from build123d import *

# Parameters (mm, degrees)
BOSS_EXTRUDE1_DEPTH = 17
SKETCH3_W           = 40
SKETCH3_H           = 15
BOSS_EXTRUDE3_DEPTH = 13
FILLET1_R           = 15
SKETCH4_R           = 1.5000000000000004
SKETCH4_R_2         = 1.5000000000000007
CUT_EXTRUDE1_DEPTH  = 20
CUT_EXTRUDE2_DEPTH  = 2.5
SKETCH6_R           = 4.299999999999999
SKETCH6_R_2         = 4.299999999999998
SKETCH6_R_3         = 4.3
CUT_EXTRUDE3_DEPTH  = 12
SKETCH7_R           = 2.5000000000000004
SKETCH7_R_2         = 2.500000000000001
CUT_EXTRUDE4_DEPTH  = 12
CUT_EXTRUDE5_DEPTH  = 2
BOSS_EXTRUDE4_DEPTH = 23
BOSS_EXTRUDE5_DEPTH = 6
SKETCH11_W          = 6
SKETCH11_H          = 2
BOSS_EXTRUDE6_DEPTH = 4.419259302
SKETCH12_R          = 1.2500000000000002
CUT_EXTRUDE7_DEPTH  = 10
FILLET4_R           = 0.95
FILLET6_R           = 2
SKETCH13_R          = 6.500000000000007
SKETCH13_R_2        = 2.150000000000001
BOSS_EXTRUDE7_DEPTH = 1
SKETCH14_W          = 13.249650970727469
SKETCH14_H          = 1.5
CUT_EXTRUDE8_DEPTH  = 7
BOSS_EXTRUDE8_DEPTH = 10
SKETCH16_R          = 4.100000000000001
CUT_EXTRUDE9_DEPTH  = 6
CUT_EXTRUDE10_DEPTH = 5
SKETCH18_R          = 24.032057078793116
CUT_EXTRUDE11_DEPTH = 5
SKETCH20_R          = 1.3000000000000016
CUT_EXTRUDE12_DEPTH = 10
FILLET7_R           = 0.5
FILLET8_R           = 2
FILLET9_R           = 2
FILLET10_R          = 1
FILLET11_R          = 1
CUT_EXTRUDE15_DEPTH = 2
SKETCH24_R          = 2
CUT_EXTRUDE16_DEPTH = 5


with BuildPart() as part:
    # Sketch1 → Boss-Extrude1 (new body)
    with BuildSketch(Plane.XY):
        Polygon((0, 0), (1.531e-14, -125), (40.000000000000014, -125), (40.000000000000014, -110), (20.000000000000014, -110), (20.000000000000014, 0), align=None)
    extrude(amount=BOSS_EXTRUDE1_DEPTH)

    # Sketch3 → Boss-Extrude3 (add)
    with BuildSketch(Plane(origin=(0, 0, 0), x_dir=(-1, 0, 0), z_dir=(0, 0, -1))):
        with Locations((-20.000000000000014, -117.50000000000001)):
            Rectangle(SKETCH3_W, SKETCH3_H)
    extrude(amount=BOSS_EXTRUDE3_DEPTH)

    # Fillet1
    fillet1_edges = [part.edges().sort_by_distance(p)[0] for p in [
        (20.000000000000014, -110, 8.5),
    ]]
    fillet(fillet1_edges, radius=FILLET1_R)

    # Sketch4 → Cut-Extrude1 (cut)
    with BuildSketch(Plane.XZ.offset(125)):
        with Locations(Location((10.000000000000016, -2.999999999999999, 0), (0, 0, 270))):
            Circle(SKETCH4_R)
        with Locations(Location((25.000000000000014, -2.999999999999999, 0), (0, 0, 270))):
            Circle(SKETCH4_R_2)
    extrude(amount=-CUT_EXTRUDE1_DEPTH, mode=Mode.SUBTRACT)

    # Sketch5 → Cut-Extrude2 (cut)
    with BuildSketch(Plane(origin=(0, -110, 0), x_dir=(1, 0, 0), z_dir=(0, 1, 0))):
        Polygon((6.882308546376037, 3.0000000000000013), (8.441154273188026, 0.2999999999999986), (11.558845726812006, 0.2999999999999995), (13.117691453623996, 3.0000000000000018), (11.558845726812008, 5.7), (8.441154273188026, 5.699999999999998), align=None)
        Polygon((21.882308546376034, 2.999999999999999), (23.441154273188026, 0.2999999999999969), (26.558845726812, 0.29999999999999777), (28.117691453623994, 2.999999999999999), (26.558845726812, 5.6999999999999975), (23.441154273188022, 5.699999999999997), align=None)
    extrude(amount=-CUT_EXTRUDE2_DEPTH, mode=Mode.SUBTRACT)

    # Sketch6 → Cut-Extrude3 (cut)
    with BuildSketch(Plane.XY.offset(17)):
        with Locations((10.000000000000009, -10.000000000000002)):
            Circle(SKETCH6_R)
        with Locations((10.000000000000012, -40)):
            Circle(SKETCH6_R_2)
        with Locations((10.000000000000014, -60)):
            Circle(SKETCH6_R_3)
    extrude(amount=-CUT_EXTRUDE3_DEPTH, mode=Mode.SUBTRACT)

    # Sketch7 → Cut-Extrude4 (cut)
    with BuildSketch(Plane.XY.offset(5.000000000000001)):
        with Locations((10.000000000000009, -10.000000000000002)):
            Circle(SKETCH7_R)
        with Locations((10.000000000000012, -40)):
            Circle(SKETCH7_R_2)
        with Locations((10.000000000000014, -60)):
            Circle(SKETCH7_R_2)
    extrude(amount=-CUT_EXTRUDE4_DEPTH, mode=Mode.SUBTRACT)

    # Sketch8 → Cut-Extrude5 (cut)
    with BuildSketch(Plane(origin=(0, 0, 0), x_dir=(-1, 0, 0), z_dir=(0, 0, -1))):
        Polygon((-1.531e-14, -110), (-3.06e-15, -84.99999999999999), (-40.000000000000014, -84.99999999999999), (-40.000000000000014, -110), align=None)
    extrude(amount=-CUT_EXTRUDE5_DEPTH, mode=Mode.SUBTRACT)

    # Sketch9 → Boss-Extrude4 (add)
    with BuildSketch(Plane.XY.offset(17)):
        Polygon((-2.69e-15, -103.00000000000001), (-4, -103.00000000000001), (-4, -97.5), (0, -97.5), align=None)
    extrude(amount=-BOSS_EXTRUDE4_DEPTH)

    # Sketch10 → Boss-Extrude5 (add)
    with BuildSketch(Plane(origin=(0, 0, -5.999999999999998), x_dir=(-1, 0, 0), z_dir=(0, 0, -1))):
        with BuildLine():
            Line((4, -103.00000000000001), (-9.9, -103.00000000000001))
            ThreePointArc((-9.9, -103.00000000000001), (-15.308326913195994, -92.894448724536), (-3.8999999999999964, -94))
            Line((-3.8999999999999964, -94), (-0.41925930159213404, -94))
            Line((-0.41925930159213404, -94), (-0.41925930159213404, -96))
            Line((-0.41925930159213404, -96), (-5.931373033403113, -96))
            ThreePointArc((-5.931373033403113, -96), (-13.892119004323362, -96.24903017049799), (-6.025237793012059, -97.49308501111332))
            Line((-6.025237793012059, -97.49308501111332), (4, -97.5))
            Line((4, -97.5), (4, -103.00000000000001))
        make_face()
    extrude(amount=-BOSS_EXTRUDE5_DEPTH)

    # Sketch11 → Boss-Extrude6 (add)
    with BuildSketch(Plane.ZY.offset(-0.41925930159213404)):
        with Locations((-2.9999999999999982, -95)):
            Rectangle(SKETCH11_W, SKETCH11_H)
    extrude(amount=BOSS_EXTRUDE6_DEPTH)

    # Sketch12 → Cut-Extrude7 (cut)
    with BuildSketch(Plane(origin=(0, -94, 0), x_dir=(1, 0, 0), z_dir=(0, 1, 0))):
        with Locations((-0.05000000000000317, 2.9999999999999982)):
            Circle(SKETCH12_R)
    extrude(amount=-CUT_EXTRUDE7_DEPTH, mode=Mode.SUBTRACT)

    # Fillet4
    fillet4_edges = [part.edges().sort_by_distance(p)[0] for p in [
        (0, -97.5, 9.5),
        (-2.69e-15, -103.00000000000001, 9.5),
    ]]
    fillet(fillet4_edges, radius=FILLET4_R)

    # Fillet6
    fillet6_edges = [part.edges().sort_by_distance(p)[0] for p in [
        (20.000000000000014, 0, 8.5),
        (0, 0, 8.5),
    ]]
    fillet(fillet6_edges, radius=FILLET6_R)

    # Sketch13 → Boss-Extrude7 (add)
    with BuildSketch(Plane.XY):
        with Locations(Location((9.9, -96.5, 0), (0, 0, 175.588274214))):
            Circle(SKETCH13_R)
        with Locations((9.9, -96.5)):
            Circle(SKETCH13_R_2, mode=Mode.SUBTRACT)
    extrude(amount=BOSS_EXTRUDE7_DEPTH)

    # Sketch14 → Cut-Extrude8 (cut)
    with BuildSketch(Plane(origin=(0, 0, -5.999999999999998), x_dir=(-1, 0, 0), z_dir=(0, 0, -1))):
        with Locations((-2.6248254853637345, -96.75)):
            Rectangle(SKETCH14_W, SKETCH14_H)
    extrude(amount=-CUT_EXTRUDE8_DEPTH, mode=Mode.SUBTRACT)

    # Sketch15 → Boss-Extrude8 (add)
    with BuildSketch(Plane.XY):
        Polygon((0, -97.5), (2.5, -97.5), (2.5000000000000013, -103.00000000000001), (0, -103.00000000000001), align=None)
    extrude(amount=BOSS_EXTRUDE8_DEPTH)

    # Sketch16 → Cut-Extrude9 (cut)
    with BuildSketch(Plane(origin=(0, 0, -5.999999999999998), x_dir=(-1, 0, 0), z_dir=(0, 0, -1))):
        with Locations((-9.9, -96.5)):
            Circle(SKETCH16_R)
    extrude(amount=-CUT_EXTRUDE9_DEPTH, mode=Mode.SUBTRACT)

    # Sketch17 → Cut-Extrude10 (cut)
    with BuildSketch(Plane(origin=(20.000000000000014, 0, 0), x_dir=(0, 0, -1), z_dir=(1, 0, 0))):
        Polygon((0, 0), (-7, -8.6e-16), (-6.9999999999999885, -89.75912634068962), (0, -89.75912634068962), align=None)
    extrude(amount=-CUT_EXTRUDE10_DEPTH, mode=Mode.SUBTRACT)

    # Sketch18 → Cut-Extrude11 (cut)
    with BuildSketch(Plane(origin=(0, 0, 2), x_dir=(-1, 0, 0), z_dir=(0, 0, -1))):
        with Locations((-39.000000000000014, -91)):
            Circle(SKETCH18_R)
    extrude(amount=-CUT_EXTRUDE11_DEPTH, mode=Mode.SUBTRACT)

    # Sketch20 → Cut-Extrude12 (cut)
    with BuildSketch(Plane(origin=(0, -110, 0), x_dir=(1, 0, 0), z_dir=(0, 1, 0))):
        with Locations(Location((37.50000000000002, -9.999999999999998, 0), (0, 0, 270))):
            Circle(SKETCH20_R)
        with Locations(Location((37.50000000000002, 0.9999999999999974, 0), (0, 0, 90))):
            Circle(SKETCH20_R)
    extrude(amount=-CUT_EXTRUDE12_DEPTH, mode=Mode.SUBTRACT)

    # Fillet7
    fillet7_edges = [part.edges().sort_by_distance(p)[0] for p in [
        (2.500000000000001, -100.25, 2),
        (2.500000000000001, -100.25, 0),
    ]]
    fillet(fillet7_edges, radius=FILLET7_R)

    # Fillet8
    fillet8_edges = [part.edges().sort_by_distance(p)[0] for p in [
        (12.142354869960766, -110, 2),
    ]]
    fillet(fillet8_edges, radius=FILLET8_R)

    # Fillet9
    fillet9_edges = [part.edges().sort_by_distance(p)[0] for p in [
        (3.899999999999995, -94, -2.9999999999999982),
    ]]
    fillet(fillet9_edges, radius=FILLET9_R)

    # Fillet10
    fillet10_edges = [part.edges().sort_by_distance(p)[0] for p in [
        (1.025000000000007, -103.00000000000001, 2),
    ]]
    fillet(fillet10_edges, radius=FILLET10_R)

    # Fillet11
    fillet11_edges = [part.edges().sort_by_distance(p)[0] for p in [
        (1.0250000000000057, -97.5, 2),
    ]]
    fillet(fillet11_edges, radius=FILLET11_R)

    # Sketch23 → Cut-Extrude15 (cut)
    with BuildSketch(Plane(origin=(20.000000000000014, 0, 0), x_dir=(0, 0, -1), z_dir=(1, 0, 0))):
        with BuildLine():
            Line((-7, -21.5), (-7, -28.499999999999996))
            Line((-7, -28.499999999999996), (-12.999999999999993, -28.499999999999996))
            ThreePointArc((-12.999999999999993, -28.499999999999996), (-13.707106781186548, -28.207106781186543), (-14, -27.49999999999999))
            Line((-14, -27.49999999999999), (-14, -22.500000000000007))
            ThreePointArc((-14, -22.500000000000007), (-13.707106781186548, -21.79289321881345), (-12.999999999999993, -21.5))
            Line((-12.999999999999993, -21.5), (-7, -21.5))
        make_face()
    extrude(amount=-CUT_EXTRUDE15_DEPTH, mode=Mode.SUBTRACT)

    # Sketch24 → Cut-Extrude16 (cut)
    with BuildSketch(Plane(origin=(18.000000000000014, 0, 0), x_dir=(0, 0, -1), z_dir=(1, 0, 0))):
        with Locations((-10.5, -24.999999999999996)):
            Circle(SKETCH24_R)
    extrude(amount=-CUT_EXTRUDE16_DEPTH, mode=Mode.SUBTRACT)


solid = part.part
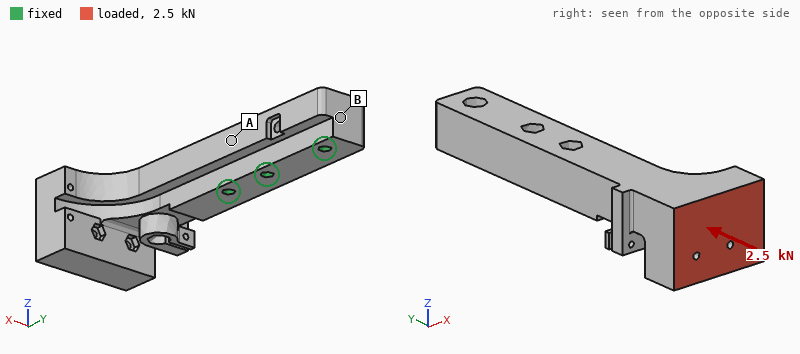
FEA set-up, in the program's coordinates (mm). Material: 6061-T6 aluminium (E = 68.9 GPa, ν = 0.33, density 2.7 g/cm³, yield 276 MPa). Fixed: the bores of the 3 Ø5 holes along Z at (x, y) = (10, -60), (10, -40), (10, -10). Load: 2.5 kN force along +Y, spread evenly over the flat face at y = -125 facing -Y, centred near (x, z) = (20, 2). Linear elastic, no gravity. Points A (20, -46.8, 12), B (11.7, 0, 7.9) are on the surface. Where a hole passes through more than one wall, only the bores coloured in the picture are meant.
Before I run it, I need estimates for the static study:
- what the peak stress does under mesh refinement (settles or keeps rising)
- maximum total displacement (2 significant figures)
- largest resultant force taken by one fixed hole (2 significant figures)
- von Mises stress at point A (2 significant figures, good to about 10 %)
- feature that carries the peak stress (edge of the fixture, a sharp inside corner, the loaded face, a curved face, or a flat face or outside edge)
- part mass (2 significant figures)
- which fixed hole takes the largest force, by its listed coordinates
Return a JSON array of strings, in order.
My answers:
["keeps rising", "0.25 mm", "2.5 kN", "16 MPa", "edge of the fixture", "130 g", "(10, -60)"]
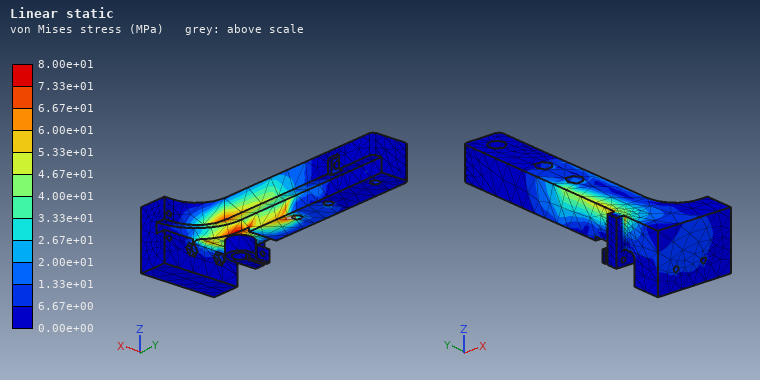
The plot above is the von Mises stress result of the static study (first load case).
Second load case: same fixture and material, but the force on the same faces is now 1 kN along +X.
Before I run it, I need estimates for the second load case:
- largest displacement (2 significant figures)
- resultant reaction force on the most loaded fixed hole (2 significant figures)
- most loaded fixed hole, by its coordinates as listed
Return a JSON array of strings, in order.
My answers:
["0.32 mm", "3.0 kN", "(10, -60)"]
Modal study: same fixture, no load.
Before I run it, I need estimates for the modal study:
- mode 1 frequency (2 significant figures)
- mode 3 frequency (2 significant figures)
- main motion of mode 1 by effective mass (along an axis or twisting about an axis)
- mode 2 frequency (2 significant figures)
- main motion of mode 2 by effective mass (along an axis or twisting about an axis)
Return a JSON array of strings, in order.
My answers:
["1300 Hz", "2900 Hz", "along Z", "1500 Hz", "along X"]
